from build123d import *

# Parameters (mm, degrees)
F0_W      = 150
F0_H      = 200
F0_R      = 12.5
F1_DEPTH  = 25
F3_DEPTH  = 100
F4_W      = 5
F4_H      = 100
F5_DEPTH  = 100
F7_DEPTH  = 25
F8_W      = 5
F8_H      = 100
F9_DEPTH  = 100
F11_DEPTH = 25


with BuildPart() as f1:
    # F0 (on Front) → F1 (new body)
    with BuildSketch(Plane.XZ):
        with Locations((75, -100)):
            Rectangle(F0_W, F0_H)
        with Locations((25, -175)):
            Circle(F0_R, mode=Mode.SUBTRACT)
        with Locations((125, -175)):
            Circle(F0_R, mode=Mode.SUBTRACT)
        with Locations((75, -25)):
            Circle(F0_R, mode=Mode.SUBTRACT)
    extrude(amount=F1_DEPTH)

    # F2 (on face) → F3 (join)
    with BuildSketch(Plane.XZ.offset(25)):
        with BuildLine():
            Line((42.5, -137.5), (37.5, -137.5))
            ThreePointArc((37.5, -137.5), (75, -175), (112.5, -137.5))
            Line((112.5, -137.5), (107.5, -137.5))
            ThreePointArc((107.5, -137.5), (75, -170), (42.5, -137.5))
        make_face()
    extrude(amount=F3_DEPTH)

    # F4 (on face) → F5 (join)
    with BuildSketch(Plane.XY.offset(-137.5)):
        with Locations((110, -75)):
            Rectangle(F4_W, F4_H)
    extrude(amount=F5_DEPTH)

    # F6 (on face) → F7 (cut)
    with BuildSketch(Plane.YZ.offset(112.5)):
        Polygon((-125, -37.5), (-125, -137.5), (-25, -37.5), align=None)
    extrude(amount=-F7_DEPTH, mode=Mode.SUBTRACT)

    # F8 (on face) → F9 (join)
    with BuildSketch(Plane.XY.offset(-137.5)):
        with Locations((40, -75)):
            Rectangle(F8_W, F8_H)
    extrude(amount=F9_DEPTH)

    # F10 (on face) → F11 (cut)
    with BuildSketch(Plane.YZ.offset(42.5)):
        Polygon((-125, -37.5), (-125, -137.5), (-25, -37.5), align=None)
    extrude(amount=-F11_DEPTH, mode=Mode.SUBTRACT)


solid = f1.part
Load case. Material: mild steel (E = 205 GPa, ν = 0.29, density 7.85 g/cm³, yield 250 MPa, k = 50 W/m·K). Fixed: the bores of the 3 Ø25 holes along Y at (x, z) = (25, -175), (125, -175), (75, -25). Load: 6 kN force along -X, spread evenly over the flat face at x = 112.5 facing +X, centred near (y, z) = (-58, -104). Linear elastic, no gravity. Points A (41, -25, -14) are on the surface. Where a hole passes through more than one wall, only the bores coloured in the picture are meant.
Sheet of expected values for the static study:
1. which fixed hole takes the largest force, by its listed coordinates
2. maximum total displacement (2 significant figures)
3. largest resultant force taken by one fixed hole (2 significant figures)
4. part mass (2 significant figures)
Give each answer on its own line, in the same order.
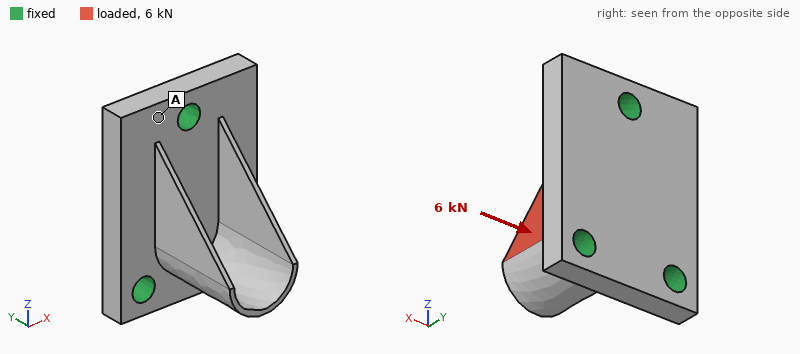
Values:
(125, -175)
0.34 mm
3.8 kN
6.4 kg
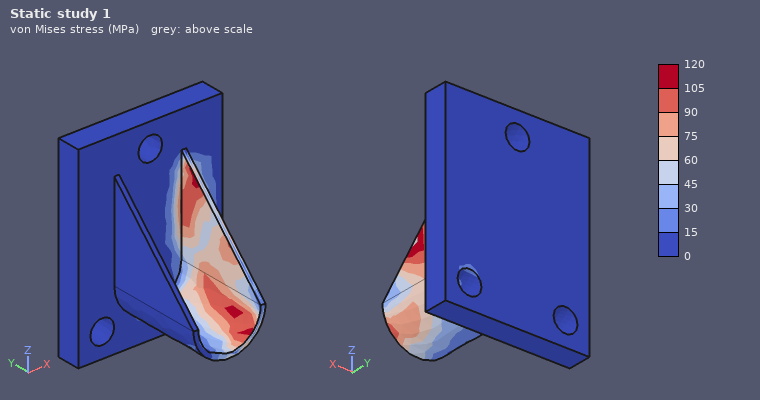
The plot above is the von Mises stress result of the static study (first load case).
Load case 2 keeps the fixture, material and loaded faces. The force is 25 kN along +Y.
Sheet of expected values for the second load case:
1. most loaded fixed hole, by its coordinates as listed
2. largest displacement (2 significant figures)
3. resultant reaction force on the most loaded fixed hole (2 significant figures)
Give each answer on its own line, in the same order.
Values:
(125, -175)
0.15 mm
14 kN
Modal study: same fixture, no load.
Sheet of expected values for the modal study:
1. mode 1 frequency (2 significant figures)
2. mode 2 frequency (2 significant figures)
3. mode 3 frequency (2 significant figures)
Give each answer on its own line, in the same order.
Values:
1700 Hz
2000 Hz
3200 Hz
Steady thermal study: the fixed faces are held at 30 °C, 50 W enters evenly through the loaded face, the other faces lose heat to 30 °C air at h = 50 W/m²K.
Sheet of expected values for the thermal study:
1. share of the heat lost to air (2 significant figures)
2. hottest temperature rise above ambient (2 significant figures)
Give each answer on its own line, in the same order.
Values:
50 %
42 K
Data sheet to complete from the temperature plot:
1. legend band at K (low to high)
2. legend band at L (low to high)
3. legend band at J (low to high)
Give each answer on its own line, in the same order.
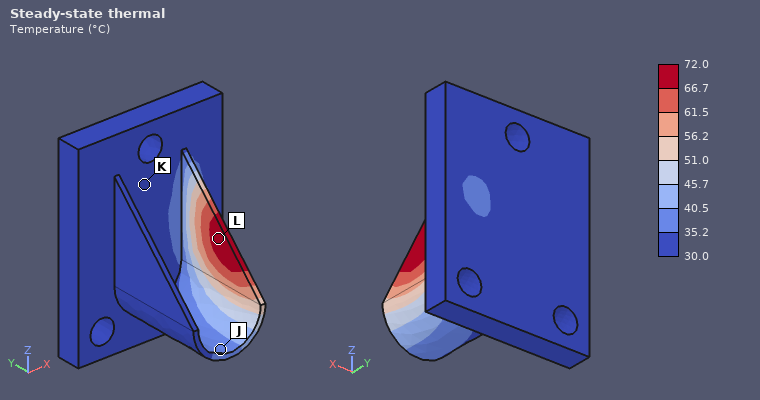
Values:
30.0 to 35.2 °C
66.7 to 72.0 °C
35.2 to 40.5 °C
